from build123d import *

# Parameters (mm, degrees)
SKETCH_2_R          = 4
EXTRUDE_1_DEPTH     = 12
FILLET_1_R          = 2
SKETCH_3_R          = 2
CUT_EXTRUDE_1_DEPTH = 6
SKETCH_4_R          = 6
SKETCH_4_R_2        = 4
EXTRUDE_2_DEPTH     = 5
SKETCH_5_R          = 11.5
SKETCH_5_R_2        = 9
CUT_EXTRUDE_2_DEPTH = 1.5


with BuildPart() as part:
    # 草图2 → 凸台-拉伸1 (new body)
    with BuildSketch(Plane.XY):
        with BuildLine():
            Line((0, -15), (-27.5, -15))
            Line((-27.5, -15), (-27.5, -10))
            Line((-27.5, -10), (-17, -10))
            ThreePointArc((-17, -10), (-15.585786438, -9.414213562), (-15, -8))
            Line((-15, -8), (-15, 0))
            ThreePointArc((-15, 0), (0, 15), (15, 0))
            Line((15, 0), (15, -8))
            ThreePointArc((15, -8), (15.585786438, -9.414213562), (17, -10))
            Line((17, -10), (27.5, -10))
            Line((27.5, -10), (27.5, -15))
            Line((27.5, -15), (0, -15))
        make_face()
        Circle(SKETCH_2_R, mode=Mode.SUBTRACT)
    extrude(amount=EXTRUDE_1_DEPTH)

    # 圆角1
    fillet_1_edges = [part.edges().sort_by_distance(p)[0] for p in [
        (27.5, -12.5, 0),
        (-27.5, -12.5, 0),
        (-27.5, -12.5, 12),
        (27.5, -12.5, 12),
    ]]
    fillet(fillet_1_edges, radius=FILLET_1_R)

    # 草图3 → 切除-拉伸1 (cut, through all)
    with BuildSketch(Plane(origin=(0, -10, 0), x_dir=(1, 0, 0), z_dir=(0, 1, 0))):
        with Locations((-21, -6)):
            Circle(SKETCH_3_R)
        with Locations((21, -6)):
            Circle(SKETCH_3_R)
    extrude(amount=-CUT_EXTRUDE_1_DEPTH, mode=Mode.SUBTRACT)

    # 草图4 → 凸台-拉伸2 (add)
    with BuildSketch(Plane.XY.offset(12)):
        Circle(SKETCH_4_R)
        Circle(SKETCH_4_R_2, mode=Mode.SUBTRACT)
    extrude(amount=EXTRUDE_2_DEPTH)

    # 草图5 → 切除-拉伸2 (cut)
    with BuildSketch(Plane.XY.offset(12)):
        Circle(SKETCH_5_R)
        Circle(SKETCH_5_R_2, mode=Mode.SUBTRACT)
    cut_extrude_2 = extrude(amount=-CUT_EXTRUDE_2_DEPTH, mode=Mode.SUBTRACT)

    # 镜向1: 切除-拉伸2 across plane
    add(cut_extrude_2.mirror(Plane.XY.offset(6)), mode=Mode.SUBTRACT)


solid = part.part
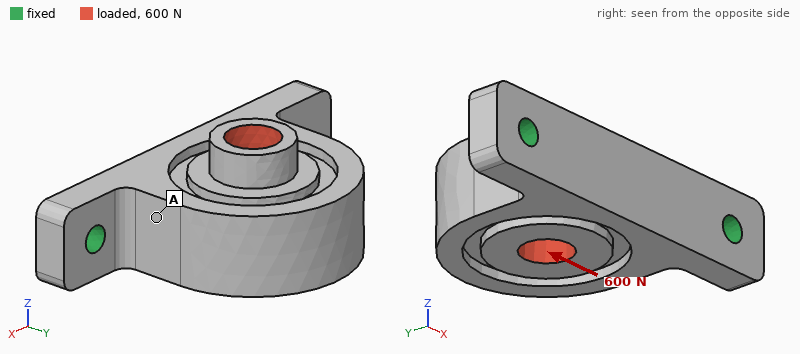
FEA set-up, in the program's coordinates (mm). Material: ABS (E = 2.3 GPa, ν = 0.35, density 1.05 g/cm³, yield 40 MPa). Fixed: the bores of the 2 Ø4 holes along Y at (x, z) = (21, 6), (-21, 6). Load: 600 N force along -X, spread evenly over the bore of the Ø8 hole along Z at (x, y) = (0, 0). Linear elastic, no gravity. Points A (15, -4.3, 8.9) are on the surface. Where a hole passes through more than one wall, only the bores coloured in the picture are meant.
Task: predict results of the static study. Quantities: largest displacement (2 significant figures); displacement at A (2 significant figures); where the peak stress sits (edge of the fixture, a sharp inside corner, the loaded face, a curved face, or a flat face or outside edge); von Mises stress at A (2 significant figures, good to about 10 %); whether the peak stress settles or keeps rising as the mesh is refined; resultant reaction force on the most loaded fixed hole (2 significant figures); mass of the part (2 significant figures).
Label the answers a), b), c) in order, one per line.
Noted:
a) 0.14 mm
b) 0.073 mm
c) edge of the fixture
d) 3.5 MPa
e) keeps rising
f) 370 N
g) 11 g
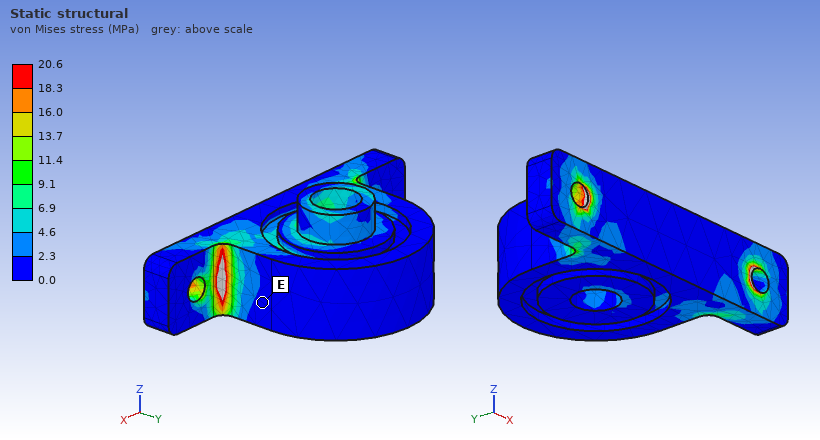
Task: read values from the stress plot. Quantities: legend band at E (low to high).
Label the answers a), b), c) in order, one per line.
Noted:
a) 0.0 to 2.3 MPa
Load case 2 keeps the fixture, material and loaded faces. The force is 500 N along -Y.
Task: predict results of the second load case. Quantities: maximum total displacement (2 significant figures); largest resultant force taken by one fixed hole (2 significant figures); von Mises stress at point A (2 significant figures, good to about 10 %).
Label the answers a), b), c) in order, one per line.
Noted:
a) 0.36 mm
b) 290 N
c) 5.4 MPa
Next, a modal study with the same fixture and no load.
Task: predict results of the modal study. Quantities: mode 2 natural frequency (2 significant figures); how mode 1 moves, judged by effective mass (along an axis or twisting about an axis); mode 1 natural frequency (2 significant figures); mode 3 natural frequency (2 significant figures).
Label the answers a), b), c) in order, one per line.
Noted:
a) 4100 Hz
b) along Z
c) 1200 Hz
d) 4200 Hz
